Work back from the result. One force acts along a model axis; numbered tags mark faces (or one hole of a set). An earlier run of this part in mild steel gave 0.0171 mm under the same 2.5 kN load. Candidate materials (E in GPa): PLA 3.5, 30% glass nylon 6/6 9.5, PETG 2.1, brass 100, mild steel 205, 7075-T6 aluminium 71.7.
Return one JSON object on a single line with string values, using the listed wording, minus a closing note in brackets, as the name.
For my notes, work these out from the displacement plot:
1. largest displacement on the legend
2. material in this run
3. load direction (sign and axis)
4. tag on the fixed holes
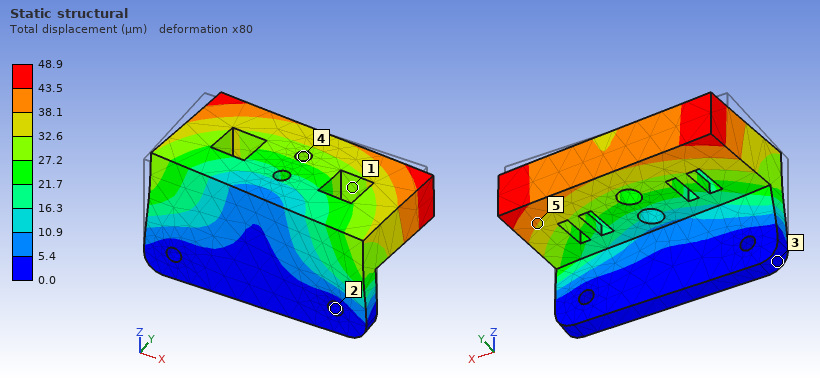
{"largest displacement on the legend": "48.9 µm", "material in this run": "7075-T6 aluminium", "load direction": "+X", "tag on the fixed holes": "2"}
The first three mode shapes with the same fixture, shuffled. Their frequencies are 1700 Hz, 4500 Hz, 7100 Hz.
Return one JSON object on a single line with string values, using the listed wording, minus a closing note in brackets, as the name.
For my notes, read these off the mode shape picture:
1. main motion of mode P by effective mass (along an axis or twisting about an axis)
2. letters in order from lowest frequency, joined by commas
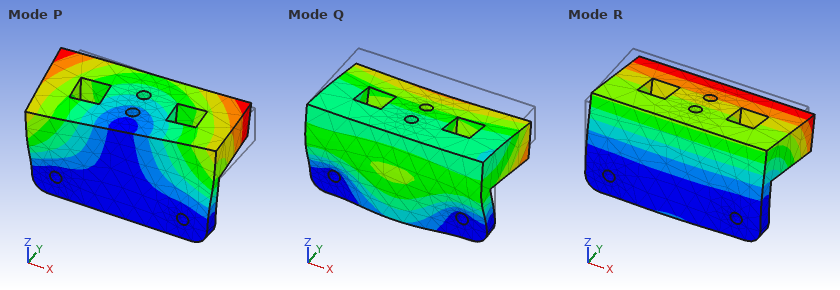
{"main motion of mode P by effective mass": "along X", "letters in order from lowest frequency, joined by commas": "R, P, Q"}
